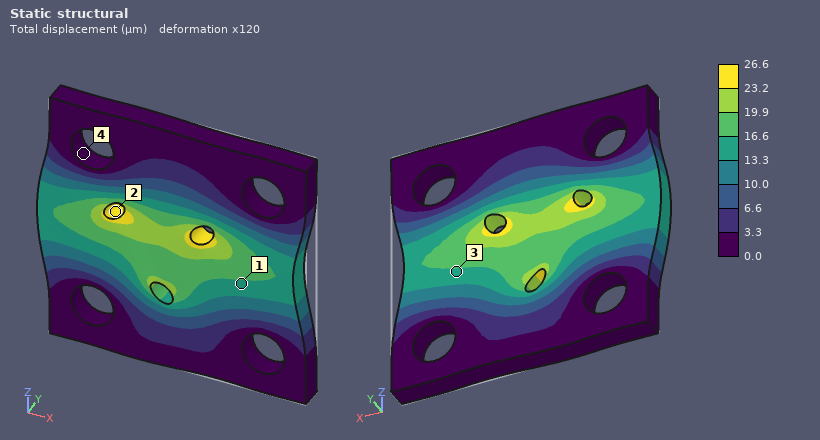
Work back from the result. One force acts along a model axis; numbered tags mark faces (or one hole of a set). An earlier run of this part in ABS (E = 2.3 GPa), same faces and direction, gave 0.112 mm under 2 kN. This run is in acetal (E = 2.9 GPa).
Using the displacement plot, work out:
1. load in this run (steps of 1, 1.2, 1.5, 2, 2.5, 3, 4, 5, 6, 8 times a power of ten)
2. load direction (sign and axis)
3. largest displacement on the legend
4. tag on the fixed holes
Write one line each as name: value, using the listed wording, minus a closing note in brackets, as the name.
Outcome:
load in this run: 600 N
load direction: -X
largest displacement on the legend: 26.6 µm
tag on the fixed holes: 4
